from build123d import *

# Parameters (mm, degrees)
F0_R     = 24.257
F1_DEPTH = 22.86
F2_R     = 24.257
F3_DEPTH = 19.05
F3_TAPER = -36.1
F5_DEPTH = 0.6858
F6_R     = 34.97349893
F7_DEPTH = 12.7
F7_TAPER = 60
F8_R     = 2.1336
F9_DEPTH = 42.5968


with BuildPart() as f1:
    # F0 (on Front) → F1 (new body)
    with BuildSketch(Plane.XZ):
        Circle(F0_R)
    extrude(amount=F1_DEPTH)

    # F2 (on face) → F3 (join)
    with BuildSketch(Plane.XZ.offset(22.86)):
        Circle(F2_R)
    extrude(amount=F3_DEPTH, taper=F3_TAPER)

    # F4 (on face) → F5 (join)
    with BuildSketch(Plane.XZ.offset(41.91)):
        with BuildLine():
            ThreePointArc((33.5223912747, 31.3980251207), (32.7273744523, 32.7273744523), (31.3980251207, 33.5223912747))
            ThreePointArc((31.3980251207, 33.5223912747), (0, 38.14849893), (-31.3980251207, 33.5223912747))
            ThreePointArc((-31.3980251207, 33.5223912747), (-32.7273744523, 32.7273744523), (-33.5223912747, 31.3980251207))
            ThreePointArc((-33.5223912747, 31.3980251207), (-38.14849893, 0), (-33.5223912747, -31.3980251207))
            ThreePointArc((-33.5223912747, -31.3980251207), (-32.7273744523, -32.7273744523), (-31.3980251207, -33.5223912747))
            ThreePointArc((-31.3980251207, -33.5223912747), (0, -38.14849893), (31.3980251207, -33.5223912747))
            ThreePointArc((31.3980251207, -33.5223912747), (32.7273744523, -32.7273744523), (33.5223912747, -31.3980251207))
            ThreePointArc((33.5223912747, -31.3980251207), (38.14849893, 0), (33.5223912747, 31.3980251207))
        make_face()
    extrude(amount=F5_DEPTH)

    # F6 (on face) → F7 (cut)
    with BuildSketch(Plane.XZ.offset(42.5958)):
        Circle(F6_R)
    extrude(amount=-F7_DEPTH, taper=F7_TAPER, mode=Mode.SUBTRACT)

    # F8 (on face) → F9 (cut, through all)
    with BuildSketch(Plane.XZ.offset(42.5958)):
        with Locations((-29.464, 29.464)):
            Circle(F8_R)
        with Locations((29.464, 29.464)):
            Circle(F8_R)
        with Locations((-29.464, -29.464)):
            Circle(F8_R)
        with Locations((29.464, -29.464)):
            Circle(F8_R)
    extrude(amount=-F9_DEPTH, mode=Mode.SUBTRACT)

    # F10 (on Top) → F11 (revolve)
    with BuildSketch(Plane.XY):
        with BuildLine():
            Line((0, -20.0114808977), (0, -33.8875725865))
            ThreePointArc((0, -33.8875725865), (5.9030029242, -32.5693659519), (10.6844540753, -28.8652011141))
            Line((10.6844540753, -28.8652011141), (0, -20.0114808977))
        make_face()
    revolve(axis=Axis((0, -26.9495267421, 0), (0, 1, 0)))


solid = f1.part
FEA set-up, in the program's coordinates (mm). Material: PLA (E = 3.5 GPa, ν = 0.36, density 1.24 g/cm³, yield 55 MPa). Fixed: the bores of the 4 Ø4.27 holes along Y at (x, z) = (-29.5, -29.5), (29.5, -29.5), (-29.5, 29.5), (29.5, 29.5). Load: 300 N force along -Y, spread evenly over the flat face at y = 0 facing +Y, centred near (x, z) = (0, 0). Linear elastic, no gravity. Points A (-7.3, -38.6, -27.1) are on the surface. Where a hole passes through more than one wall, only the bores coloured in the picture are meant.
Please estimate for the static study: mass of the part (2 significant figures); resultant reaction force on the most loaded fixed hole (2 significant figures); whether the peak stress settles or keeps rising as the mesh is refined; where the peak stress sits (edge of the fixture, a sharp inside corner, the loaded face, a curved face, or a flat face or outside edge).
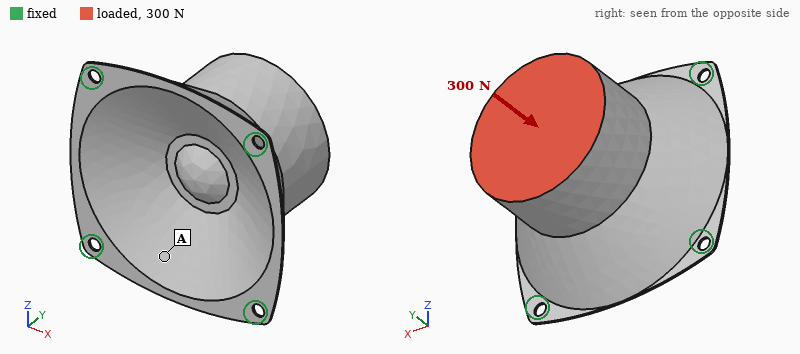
100 g
120 N
keeps rising
edge of the fixture
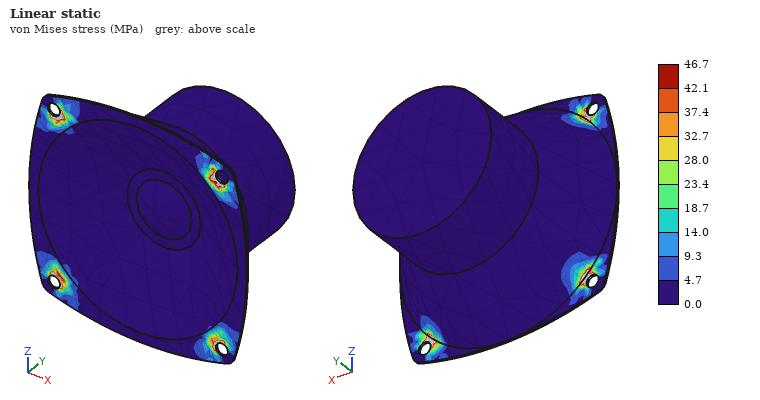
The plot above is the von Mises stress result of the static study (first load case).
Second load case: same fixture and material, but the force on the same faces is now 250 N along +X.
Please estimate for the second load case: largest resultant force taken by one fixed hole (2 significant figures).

140 N
